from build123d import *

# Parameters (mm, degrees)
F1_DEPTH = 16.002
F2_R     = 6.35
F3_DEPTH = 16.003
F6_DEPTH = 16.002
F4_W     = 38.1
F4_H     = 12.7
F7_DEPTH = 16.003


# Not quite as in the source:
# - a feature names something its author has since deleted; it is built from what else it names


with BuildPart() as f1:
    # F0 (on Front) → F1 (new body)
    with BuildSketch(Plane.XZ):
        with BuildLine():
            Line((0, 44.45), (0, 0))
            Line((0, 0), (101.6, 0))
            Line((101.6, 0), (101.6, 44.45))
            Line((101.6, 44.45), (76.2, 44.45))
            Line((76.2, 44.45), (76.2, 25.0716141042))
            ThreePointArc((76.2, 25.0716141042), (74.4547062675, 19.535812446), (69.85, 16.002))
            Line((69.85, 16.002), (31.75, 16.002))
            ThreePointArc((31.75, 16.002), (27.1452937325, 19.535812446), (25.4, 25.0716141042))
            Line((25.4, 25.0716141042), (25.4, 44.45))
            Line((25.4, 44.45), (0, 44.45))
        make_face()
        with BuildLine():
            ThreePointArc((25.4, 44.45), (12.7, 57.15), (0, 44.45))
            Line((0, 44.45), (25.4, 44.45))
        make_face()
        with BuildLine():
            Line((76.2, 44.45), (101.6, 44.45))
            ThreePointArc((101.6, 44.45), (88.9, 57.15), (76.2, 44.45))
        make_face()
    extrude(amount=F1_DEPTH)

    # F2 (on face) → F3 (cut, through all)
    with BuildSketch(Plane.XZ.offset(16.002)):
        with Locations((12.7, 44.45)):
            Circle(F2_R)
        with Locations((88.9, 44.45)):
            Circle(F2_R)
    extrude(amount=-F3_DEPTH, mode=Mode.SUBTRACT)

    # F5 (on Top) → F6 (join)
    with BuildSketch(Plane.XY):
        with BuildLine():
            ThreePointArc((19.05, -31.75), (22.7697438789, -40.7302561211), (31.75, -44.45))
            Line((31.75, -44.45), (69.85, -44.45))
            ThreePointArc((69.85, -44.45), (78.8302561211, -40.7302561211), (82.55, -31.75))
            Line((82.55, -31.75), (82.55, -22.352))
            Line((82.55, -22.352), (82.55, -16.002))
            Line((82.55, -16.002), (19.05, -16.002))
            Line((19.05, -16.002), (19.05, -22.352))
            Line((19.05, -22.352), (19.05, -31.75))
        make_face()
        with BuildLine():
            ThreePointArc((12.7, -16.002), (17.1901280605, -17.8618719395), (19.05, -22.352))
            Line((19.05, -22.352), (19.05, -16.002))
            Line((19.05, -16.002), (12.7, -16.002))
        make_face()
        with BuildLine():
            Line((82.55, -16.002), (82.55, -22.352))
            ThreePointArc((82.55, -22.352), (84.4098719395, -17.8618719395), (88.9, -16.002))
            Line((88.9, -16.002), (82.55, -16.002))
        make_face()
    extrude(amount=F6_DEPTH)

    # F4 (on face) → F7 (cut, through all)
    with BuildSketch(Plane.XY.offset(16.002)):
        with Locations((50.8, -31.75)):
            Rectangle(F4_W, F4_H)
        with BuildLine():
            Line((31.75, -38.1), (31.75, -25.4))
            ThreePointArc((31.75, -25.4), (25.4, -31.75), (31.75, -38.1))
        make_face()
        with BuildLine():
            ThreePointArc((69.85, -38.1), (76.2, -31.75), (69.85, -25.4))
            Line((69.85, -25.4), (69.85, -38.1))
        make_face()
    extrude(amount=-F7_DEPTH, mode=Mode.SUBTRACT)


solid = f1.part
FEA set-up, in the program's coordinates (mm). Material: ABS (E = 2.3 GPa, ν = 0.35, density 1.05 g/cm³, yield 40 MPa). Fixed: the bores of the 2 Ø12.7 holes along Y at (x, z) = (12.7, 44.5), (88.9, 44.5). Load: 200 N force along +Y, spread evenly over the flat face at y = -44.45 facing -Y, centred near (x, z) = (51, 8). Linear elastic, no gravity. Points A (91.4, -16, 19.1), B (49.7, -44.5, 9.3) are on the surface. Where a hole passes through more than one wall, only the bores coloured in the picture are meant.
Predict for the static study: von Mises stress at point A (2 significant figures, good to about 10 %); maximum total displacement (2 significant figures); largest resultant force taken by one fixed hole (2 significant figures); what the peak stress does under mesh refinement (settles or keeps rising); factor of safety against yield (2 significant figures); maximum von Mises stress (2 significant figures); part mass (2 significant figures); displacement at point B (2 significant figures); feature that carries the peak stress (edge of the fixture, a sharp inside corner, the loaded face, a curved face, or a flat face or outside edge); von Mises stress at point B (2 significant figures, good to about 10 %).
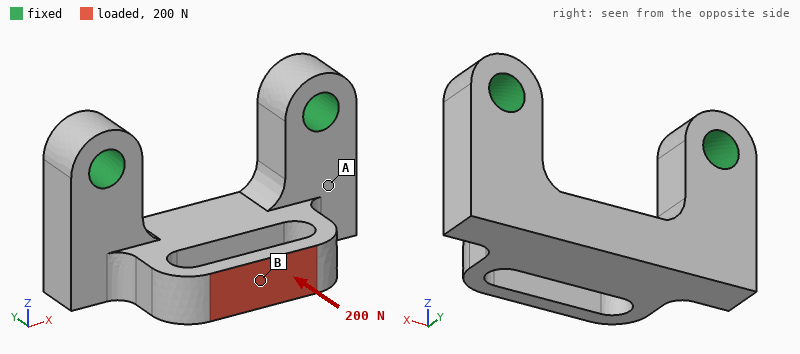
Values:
1.0 MPa
0.32 mm
100 N
settles
4.4
9.2 MPa
76 g
0.29 mm
a curved face
6.9 MPa
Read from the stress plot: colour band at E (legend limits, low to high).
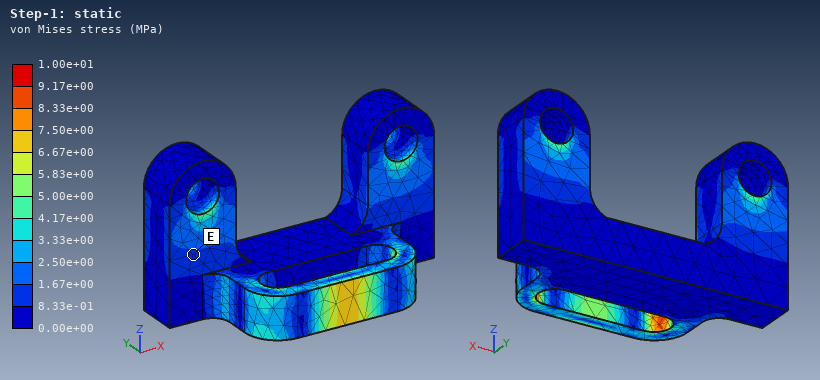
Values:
8.33e-01 to 1.67e+00 MPa
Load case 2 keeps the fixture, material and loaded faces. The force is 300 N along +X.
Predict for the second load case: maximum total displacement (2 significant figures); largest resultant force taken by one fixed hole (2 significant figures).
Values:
0.26 mm
210 N
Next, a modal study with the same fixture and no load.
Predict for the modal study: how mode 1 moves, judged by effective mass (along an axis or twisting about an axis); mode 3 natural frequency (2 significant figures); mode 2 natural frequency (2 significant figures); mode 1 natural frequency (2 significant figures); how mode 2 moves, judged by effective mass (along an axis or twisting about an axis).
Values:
along Y
2000 Hz
1700 Hz
970 Hz
along X
